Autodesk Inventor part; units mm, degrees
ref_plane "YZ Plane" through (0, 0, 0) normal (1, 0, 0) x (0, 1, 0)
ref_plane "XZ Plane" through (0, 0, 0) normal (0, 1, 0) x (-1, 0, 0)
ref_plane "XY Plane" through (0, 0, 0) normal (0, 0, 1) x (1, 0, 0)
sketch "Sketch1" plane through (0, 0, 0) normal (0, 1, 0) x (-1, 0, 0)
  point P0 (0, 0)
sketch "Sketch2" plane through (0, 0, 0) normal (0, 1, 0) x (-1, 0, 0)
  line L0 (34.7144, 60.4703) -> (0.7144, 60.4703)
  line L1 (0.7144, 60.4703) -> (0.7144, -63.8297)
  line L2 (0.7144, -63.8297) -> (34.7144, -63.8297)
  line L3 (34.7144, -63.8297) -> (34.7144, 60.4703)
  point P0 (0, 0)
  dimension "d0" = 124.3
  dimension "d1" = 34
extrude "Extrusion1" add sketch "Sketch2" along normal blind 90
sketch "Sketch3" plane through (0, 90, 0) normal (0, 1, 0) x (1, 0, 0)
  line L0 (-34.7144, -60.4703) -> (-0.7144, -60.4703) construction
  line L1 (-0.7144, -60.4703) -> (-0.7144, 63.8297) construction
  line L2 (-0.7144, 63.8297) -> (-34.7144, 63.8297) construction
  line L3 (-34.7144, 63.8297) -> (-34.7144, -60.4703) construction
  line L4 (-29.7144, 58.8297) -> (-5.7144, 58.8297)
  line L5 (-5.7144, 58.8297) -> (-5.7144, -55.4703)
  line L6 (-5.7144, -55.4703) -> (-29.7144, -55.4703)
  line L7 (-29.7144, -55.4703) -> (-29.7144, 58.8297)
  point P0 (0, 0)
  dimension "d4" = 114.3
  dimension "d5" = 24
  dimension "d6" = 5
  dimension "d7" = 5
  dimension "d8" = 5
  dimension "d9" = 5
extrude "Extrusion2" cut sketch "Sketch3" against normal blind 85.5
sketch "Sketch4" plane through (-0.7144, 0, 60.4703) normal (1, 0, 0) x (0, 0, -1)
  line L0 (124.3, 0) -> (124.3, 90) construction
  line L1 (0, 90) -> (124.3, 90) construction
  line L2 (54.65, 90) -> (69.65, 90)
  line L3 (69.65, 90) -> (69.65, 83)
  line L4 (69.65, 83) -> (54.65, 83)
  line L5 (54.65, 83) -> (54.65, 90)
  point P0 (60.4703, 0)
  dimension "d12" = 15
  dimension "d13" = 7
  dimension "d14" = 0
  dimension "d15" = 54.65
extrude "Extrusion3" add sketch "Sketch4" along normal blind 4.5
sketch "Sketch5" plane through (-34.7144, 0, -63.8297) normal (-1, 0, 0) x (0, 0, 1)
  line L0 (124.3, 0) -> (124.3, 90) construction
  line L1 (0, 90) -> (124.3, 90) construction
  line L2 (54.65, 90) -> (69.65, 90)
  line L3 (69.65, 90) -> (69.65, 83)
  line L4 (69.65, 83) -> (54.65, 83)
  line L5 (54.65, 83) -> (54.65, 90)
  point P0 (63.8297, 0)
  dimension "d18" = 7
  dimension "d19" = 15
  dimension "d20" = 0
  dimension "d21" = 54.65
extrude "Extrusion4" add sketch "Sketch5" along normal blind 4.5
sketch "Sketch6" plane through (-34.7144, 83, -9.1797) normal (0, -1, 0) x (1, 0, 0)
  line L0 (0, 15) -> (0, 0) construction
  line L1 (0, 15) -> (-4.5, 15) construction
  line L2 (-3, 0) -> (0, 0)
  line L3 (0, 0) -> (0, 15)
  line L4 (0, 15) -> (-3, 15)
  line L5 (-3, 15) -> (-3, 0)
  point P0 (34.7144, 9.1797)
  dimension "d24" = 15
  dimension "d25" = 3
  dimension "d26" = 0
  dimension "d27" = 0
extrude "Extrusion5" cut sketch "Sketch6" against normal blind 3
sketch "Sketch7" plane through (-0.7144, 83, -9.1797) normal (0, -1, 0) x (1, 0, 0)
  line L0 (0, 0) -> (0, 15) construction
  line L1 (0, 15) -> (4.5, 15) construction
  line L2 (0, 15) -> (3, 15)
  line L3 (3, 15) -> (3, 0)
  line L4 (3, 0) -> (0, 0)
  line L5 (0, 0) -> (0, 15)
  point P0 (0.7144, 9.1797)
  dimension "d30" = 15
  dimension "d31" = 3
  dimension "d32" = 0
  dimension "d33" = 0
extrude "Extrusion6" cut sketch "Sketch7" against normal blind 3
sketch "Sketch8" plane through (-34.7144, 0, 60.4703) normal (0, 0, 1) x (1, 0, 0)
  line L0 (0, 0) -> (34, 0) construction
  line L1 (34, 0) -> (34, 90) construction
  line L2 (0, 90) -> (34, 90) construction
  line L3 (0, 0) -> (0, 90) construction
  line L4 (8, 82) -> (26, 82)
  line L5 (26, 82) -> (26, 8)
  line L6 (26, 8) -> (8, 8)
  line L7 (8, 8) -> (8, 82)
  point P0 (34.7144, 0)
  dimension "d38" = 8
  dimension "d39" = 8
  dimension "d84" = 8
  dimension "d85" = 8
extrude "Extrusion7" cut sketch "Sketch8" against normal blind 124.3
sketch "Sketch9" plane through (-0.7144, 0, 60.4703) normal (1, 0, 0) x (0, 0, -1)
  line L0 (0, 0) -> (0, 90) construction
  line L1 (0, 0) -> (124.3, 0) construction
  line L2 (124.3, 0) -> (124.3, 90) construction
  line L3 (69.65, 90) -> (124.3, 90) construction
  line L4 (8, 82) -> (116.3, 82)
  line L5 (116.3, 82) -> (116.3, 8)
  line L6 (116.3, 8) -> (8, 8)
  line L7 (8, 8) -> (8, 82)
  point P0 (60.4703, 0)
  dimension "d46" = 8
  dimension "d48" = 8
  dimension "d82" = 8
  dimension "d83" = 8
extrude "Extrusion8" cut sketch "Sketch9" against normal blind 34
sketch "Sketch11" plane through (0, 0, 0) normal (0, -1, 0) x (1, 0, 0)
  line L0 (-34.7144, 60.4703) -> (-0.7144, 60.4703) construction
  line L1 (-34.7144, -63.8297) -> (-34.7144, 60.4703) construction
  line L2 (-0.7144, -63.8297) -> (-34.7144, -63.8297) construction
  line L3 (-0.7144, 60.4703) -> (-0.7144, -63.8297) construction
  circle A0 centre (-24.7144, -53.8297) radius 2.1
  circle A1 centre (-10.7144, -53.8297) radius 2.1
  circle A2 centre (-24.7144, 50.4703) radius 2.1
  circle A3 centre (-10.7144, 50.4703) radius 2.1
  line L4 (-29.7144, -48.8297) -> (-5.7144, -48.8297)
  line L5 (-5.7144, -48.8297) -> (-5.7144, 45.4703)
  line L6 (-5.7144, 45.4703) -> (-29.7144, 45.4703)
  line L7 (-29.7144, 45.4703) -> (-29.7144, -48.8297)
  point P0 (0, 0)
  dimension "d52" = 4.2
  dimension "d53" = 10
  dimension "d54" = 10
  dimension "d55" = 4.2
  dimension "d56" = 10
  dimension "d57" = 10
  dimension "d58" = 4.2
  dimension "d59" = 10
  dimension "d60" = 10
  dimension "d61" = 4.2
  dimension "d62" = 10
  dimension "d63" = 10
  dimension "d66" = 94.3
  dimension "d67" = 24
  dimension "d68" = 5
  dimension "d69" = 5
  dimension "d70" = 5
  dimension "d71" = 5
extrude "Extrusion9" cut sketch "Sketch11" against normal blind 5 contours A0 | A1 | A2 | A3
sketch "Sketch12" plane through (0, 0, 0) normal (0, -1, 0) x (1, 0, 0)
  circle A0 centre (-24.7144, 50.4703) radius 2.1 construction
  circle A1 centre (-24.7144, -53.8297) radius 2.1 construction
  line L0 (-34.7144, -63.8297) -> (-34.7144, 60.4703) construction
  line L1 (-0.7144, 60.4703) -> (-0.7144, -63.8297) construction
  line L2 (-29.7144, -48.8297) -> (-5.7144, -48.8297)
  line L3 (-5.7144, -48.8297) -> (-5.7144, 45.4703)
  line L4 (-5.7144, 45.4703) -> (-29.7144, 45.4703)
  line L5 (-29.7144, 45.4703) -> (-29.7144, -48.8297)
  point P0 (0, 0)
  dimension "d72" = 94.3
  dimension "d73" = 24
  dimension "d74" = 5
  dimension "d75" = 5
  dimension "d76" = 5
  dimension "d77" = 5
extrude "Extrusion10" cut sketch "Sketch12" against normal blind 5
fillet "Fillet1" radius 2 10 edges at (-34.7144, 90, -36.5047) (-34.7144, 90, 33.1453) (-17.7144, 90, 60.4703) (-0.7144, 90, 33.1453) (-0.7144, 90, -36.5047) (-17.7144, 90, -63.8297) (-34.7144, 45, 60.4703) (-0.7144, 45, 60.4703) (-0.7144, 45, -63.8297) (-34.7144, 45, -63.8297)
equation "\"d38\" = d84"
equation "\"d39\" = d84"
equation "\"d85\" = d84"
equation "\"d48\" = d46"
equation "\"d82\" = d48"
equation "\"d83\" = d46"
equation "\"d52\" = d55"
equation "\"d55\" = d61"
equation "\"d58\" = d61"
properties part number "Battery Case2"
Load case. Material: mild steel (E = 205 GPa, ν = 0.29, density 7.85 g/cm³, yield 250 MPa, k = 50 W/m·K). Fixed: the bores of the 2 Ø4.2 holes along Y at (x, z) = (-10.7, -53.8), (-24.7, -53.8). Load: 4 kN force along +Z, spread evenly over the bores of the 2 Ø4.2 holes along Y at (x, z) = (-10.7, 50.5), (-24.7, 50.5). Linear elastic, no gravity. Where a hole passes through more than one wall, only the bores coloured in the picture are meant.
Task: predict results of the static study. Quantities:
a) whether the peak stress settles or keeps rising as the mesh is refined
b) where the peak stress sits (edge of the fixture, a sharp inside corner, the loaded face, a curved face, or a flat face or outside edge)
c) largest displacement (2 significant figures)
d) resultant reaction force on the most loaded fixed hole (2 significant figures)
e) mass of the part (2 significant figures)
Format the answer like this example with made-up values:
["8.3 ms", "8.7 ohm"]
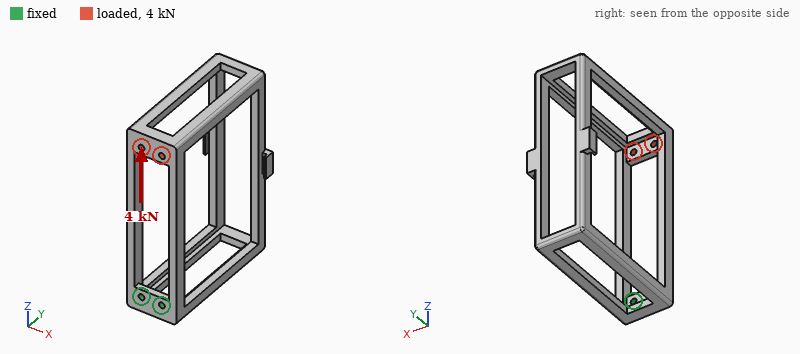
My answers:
["keeps rising", "edge of the fixture", "0.18 mm", "2.2 kN", "330 g"]
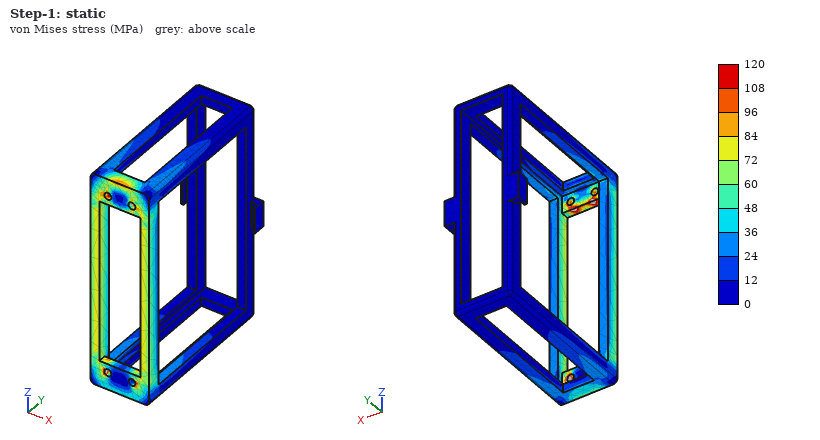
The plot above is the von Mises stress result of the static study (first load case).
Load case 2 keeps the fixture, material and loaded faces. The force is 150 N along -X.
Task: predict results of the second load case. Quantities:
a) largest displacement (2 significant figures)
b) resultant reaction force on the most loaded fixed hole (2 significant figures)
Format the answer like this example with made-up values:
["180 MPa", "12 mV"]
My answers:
["0.39 mm", "730 N"]
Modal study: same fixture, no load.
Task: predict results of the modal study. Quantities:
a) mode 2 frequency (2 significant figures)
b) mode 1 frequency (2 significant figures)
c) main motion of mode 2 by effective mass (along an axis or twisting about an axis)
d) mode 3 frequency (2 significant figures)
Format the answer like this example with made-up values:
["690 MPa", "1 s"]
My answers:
["240 Hz", "220 Hz", "along X", "470 Hz"]
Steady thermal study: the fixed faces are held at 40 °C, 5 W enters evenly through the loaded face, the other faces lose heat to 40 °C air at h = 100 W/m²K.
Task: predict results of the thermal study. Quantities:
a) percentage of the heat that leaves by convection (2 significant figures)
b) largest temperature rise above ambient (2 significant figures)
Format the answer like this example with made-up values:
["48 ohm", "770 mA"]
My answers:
["99 %", "16 K"]
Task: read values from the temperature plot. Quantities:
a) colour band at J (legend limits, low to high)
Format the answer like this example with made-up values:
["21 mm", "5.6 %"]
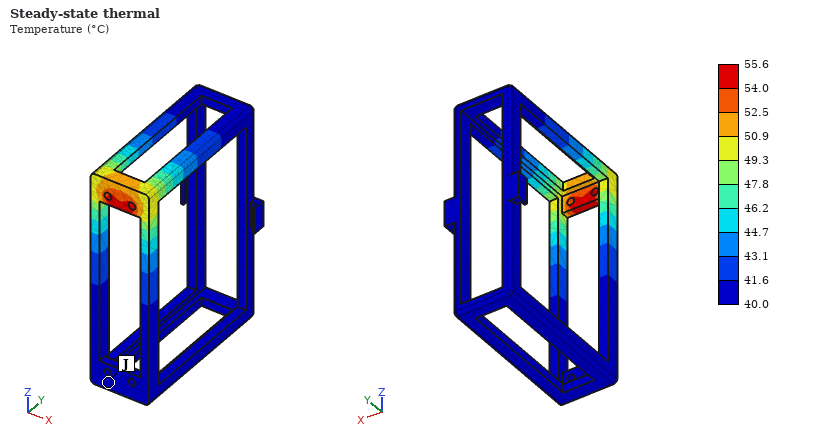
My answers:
["40.0 to 41.6 °C"]
